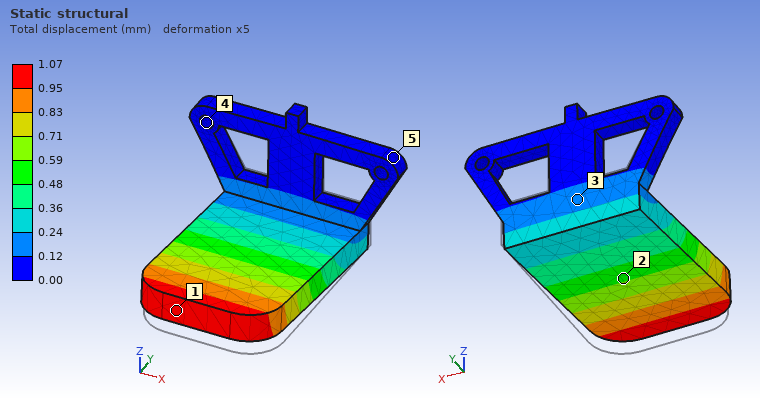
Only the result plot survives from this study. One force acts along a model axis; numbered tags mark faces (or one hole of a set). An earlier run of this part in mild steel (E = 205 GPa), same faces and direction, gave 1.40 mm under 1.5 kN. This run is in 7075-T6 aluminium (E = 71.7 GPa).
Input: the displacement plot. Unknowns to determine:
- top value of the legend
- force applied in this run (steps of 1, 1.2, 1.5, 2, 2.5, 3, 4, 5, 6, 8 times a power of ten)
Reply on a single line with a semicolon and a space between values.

1.07 mm; 400 N
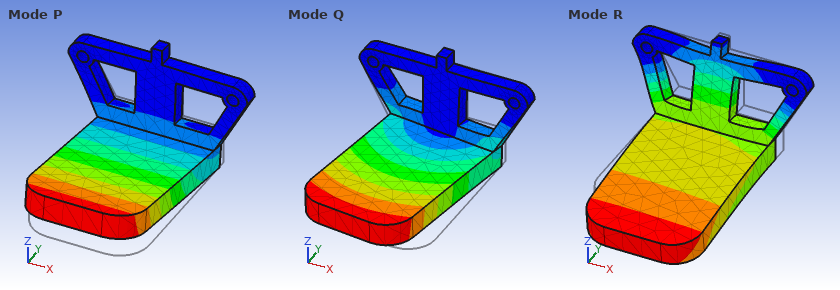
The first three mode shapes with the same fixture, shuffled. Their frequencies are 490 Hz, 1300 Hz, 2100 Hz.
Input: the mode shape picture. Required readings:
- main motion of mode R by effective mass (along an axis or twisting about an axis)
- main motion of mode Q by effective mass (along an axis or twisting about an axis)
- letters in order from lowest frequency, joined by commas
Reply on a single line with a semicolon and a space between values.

along Y; along X; P, Q, R
